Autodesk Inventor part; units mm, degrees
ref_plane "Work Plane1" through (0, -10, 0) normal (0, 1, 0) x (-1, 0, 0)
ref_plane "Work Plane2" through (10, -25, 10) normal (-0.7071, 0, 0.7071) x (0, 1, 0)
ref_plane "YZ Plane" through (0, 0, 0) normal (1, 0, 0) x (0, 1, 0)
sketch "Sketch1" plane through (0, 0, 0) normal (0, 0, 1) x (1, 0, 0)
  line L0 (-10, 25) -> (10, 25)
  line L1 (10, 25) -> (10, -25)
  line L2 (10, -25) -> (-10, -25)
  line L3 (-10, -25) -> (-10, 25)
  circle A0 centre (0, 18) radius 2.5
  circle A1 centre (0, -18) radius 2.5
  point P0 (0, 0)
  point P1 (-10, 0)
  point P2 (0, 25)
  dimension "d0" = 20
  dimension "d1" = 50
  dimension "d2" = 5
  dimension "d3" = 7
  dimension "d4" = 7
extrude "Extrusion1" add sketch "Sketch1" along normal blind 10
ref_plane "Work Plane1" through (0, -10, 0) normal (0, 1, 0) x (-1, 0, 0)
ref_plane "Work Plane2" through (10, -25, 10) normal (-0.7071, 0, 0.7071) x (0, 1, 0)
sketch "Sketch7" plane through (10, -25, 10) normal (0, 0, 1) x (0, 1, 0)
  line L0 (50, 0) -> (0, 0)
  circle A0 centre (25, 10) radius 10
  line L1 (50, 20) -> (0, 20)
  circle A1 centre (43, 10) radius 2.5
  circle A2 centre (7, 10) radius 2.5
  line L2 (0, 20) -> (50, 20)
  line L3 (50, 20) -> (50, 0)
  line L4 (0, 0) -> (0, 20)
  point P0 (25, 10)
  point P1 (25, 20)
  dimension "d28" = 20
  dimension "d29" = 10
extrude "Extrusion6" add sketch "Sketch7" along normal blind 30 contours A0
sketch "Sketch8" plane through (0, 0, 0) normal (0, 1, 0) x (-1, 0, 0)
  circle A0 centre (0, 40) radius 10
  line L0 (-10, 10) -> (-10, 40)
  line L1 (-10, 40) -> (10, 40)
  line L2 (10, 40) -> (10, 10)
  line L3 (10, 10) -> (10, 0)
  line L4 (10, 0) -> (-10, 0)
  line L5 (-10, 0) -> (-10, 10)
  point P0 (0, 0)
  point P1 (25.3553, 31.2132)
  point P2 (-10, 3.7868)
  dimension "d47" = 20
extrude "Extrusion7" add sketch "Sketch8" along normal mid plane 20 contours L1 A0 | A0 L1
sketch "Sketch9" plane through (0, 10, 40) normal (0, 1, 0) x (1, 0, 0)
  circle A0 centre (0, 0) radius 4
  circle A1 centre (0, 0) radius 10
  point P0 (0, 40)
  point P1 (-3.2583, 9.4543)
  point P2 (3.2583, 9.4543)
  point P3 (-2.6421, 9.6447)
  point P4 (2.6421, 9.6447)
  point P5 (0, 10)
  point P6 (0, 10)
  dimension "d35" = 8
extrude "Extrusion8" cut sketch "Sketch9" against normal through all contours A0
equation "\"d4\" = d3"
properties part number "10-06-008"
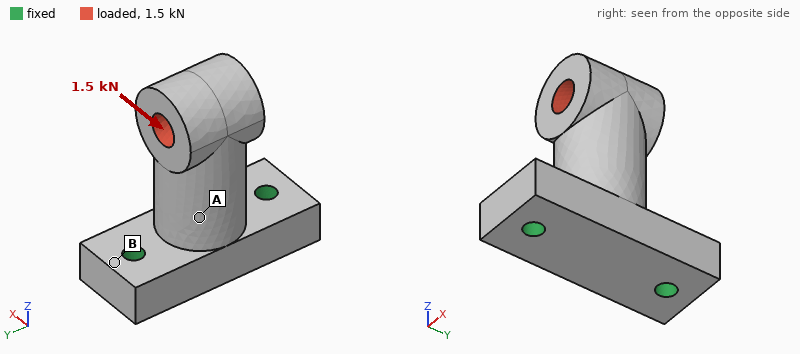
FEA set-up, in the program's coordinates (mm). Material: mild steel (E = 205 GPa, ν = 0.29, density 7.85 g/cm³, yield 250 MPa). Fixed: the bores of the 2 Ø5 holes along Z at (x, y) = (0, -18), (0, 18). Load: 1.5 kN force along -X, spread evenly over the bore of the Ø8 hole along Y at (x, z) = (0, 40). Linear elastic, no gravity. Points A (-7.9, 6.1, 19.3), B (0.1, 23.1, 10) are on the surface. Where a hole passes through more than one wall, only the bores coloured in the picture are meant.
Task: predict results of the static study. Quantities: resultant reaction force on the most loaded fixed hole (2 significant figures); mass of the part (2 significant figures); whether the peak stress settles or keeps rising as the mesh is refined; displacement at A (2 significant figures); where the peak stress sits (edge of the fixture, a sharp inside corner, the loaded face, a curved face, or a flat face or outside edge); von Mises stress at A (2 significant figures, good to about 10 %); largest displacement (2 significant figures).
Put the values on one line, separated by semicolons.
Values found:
750 N; 170 g; keeps rising; 18 µm; edge of the fixture; 32 MPa; 57 µm
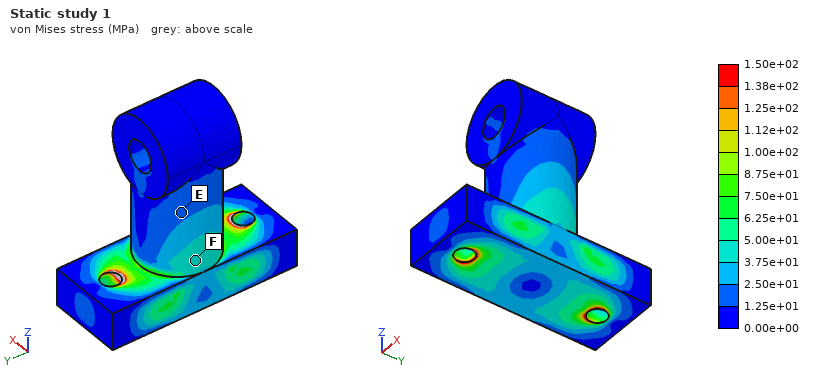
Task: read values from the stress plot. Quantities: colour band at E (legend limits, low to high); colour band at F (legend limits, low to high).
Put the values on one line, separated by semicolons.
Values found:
1.25e+01 to 2.50e+01 MPa; 3.75e+01 to 5.00e+01 MPa
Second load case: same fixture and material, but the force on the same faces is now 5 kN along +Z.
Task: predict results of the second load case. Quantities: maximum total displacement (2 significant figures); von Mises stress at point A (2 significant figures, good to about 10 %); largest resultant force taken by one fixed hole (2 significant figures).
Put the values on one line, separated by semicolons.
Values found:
7.0 µm; 15 MPa; 2.6 kN
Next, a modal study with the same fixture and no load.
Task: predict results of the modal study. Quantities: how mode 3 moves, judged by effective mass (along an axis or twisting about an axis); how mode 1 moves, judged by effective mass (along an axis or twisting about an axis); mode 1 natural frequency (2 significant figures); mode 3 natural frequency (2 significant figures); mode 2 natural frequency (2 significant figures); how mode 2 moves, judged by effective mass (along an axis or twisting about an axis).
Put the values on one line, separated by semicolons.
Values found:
along Z; along X; 4000 Hz; 15 kHz; 6300 Hz; along Y
